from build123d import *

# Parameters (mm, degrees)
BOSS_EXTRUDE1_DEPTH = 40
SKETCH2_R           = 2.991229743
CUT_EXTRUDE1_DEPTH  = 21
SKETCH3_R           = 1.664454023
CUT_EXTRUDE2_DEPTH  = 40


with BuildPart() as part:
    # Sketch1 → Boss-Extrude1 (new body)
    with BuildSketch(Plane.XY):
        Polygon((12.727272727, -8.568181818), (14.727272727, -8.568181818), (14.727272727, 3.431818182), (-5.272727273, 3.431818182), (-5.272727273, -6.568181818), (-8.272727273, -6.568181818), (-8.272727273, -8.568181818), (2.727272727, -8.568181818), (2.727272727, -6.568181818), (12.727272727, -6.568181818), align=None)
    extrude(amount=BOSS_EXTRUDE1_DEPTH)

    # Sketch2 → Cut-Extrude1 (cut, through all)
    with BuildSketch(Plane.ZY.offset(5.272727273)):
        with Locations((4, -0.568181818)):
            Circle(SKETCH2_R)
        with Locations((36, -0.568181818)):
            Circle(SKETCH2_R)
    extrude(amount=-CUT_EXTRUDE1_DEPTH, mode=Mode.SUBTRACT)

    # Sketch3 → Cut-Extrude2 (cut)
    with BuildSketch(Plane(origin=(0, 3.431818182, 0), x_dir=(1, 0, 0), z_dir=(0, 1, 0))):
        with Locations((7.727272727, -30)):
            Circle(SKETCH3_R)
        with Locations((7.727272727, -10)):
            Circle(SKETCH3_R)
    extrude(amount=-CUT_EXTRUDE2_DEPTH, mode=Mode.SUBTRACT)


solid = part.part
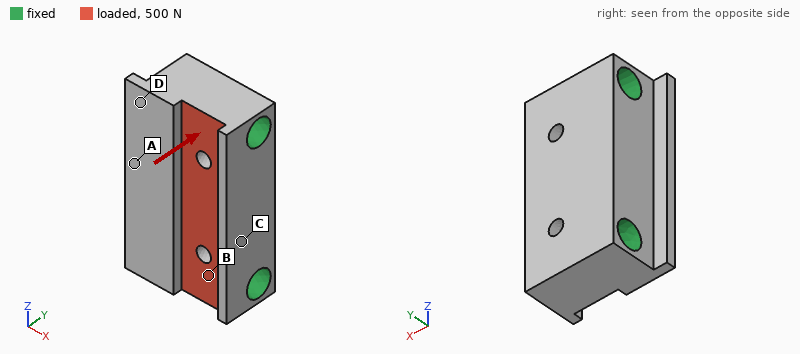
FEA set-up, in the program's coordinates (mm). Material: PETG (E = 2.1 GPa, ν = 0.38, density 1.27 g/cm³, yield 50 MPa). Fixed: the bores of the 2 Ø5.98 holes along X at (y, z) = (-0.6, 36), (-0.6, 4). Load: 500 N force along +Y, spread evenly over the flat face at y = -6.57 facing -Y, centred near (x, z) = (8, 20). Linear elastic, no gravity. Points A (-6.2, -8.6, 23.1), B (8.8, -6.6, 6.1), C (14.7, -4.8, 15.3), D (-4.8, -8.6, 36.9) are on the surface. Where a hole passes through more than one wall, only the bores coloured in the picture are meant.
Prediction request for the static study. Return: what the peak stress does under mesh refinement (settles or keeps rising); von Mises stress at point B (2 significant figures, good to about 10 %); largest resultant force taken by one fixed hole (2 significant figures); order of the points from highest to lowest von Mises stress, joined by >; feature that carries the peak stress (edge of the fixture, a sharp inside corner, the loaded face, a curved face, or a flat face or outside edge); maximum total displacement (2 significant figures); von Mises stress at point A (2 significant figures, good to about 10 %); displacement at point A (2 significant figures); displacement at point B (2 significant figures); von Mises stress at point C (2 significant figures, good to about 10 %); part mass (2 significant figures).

keeps rising
2.3 MPa
260 N
B > C > A > D
edge of the fixture
25 µm
0.86 MPa
6.3 µm
5.1 µm
1.4 MPa
9.8 g
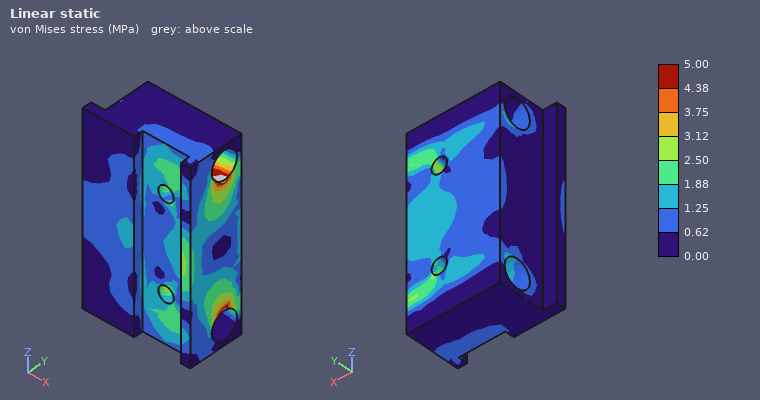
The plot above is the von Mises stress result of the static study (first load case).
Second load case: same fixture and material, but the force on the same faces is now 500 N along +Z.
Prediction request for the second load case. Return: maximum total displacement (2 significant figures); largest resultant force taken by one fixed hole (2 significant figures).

12 µm
260 N
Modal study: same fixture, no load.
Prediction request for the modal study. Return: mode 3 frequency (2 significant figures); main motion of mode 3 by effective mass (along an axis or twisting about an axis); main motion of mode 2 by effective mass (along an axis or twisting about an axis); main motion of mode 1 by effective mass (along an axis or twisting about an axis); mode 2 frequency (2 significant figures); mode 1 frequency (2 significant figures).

11 kHz
along X
along X
along Y
10 kHz
9200 Hz
